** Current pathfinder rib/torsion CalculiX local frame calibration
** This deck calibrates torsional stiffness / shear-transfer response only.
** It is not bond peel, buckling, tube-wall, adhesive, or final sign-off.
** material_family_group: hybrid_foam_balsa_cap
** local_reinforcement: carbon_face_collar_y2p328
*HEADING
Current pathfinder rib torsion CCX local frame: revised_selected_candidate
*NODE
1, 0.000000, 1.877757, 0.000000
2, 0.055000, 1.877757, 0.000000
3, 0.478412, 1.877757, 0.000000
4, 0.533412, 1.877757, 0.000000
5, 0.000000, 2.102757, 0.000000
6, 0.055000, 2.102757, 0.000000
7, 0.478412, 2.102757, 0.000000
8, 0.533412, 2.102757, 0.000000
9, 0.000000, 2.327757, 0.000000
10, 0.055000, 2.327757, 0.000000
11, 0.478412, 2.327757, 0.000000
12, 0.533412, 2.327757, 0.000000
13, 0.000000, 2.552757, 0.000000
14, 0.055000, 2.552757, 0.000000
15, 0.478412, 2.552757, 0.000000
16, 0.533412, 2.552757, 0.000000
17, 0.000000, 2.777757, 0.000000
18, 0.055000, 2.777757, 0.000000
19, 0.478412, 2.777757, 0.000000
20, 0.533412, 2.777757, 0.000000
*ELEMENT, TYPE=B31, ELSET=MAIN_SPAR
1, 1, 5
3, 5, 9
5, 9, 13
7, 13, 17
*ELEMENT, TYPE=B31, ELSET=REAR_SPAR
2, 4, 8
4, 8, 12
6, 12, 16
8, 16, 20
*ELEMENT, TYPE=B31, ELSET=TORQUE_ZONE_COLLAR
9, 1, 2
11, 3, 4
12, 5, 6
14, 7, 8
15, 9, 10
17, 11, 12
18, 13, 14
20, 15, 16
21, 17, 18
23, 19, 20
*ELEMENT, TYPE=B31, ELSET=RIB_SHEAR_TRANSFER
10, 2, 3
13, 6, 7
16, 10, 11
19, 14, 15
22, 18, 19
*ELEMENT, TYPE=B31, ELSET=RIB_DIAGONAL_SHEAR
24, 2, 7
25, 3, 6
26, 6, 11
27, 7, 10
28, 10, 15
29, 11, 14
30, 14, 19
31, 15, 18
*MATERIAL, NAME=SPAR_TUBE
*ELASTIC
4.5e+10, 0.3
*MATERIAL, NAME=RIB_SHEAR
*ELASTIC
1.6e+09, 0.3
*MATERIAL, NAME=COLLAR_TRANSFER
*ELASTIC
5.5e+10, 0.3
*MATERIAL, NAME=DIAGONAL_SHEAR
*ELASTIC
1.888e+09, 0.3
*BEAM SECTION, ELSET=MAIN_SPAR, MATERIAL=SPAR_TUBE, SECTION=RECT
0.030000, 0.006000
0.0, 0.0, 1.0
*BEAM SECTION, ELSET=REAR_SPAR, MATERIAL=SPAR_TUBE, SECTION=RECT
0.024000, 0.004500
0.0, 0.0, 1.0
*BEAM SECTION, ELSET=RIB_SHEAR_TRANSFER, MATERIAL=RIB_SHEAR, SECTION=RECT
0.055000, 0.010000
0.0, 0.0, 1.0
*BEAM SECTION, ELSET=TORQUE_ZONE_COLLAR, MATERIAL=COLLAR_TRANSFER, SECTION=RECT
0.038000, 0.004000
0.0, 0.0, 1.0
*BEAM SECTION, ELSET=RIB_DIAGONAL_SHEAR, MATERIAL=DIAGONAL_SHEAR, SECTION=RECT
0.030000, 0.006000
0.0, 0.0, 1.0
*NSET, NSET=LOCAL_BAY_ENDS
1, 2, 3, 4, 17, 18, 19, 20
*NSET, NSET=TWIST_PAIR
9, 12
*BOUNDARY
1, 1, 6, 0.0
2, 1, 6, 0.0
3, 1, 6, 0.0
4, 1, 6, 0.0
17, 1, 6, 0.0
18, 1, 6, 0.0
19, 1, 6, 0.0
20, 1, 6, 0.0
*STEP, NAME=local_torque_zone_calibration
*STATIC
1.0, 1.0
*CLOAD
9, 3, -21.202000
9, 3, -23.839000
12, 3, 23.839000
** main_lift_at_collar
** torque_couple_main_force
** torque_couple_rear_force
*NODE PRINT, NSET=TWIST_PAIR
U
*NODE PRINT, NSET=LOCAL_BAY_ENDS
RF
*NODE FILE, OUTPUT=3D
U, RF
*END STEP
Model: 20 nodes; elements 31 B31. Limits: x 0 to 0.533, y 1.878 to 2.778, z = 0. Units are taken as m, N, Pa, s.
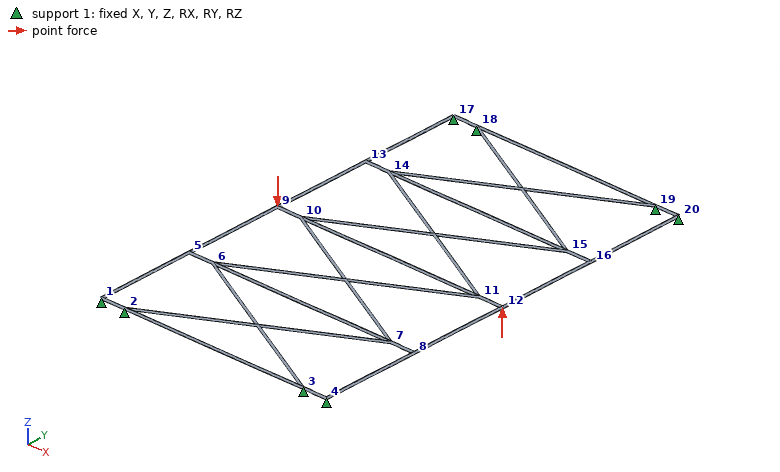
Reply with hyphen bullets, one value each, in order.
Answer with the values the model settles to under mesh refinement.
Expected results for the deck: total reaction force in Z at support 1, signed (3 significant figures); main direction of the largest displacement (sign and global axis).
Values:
- 21.2 N
- +Z
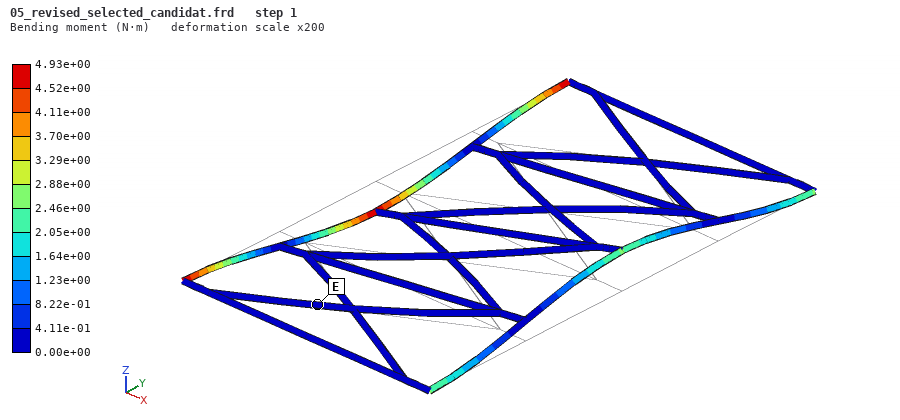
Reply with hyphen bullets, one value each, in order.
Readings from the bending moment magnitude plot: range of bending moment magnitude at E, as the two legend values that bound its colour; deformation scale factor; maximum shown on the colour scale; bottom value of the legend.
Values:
- 0.00e+00 to 4.11e-01 N·m
- 200
- 4.93e+00 N·m
- 0.00e+00 N·m
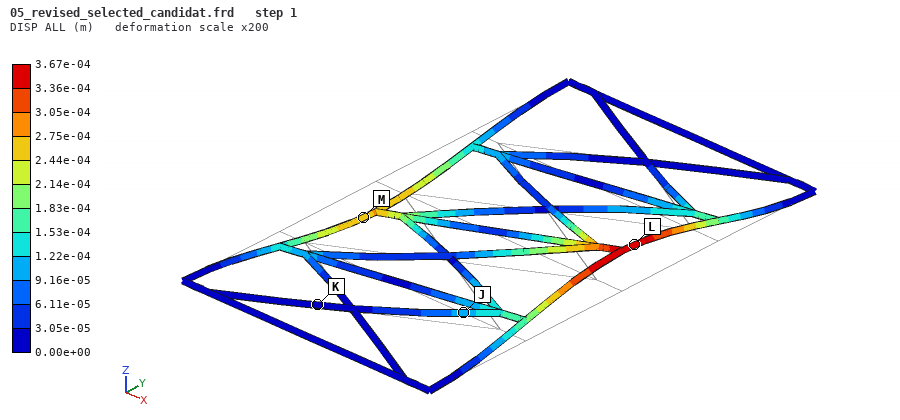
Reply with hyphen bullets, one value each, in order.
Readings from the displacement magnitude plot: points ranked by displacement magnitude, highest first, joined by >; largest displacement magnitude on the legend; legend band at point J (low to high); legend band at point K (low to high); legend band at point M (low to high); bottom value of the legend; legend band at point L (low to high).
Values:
- L > M > J > K
- 3.67e-04 m
- 9.16e-05 to 1.22e-04 m
- 0.00e+00 to 3.05e-05 m
- 2.44e-04 to 2.75e-04 m
- 0.00e+00 m
- 3.36e-04 to 3.67e-04 m
